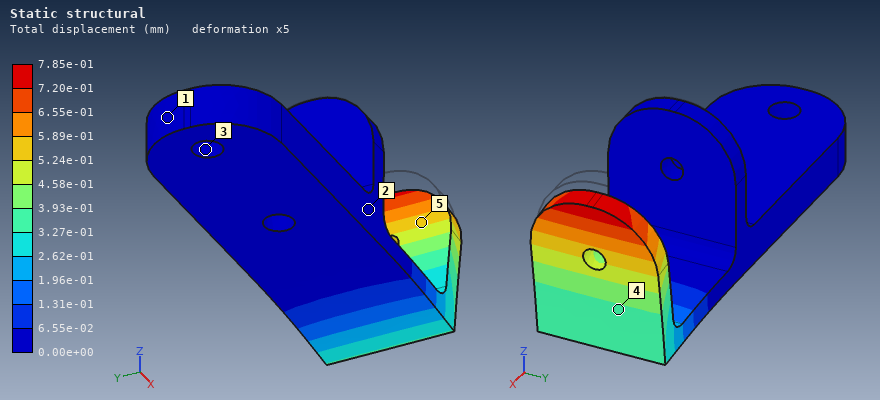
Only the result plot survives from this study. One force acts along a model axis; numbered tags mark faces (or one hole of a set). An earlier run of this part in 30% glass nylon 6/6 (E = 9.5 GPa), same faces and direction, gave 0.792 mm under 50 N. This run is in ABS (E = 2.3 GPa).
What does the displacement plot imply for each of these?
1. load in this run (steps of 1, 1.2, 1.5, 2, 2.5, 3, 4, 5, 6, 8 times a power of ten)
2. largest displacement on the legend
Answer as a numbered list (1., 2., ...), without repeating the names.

1. 12 N
2. 7.85e-01 mm
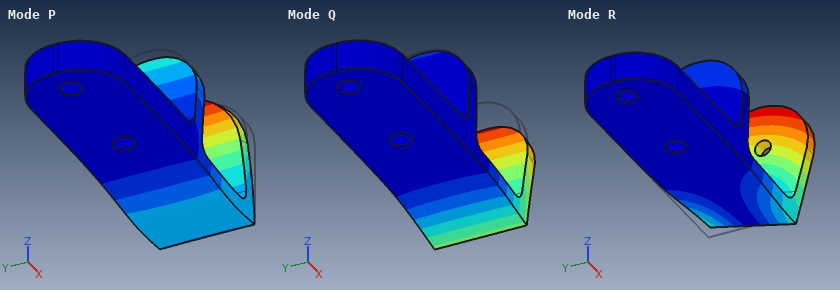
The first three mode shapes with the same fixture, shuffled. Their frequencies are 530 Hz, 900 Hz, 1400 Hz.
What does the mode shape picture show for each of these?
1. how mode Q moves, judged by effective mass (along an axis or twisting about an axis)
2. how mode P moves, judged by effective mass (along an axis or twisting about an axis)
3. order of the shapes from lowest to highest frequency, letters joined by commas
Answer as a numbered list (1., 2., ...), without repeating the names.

1. along Z
2. along Z
3. Q, R, P
